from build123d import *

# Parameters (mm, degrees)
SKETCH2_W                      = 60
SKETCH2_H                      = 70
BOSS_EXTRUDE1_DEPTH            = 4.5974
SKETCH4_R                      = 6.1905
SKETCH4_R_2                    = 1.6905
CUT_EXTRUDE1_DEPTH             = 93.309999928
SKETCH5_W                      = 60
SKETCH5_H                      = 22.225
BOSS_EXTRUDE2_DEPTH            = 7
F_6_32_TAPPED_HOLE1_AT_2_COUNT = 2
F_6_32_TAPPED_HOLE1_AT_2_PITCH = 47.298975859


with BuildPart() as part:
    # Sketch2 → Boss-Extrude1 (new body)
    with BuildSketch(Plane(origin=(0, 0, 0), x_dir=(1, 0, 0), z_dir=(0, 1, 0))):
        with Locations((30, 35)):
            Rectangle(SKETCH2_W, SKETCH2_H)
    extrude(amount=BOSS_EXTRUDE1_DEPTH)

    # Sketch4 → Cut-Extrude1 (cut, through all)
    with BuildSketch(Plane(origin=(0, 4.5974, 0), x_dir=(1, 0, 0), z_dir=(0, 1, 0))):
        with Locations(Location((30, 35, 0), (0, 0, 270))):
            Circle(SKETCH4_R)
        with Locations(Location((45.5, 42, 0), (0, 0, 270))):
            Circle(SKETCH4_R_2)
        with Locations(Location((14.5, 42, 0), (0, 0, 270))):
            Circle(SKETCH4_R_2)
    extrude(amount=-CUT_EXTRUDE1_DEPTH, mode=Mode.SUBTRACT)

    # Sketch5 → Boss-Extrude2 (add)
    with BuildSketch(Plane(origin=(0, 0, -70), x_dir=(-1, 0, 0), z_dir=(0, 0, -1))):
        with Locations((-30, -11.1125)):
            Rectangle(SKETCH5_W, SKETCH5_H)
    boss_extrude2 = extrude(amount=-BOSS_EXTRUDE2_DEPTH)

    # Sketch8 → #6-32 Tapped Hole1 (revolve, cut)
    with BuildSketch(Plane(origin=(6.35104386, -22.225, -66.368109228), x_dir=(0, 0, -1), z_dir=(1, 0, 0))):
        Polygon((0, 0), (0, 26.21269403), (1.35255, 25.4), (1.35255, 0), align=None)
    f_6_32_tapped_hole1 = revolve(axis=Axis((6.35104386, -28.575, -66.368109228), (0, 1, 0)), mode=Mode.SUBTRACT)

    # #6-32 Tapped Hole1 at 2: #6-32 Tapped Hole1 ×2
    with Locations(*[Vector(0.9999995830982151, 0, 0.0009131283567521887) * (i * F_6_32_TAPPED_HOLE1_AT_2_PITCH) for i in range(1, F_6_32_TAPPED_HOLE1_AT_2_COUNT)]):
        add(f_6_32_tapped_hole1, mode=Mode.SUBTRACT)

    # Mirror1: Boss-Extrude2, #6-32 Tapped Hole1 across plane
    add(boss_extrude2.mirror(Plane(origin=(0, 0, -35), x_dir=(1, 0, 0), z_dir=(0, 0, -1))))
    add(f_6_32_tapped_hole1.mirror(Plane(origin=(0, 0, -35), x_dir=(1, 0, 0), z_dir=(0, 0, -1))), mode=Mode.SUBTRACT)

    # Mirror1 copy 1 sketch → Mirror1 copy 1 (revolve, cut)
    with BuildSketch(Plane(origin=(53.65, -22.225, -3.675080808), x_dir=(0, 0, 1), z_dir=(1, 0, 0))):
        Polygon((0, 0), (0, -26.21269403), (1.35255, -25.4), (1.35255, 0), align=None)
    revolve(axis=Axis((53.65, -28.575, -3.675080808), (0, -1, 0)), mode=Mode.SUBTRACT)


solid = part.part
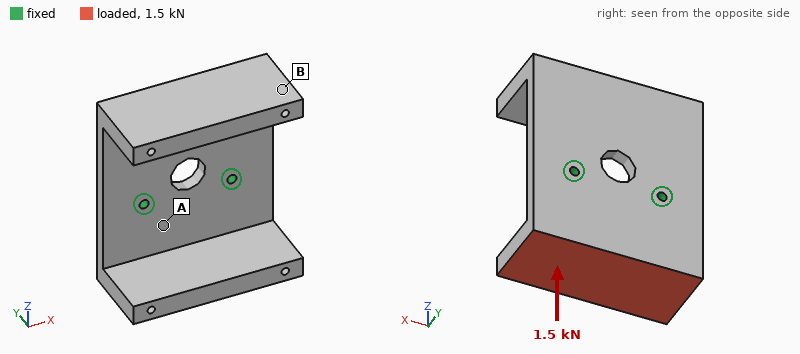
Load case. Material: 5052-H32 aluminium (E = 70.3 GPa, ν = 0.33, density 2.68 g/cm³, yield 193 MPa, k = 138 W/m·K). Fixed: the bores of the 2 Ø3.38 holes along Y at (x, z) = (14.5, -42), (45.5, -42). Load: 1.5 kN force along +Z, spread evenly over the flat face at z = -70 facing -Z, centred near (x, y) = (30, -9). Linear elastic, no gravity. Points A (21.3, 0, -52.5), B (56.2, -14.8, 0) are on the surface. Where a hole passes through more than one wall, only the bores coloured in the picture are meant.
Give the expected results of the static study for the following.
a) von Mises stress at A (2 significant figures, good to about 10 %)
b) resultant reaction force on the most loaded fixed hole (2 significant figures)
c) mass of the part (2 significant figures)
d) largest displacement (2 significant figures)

76 MPa
760 N
98 g
0.38 mm
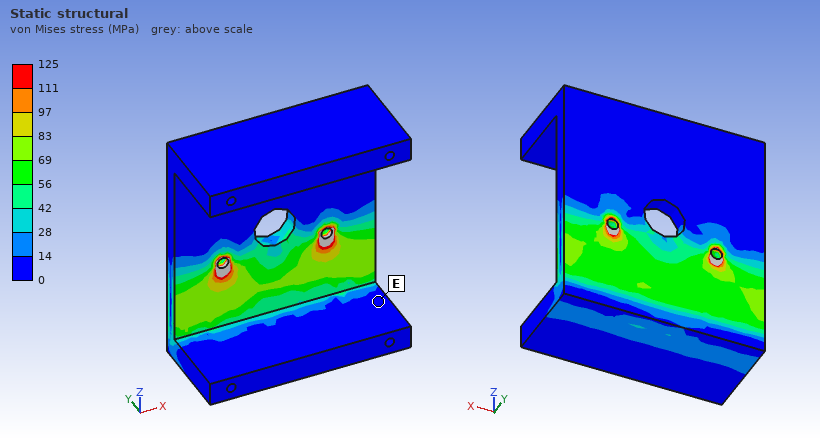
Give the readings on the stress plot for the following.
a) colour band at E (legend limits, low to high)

0 to 14 MPa
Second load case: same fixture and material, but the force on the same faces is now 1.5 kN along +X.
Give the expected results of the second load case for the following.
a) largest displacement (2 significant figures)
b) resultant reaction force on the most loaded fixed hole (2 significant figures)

0.10 mm
1.5 kN
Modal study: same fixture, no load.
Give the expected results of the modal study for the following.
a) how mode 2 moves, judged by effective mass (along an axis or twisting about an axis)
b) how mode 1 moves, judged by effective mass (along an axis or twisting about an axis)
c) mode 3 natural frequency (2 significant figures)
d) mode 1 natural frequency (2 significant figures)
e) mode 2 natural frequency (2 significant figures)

along Y
along Y
2000 Hz
920 Hz
1700 Hz
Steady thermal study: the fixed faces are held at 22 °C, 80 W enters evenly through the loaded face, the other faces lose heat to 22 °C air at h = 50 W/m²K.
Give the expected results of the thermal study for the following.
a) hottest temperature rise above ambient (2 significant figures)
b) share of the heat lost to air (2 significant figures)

64 K
19 %
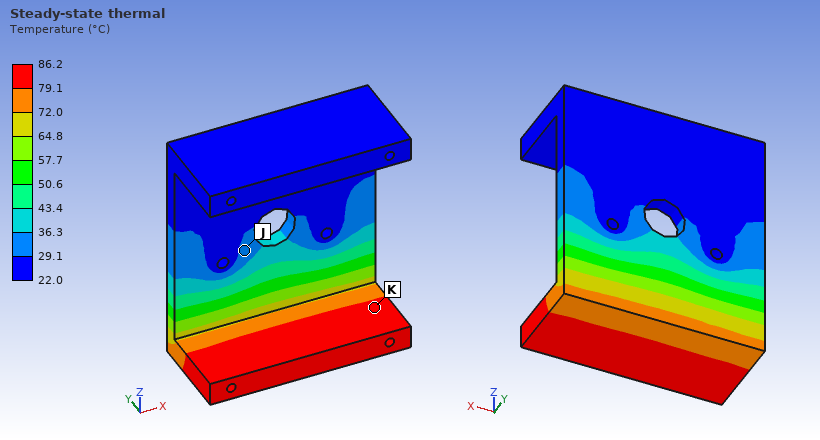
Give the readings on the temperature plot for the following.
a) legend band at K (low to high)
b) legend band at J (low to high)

79.1 to 86.2 °C
29.1 to 36.3 °C
